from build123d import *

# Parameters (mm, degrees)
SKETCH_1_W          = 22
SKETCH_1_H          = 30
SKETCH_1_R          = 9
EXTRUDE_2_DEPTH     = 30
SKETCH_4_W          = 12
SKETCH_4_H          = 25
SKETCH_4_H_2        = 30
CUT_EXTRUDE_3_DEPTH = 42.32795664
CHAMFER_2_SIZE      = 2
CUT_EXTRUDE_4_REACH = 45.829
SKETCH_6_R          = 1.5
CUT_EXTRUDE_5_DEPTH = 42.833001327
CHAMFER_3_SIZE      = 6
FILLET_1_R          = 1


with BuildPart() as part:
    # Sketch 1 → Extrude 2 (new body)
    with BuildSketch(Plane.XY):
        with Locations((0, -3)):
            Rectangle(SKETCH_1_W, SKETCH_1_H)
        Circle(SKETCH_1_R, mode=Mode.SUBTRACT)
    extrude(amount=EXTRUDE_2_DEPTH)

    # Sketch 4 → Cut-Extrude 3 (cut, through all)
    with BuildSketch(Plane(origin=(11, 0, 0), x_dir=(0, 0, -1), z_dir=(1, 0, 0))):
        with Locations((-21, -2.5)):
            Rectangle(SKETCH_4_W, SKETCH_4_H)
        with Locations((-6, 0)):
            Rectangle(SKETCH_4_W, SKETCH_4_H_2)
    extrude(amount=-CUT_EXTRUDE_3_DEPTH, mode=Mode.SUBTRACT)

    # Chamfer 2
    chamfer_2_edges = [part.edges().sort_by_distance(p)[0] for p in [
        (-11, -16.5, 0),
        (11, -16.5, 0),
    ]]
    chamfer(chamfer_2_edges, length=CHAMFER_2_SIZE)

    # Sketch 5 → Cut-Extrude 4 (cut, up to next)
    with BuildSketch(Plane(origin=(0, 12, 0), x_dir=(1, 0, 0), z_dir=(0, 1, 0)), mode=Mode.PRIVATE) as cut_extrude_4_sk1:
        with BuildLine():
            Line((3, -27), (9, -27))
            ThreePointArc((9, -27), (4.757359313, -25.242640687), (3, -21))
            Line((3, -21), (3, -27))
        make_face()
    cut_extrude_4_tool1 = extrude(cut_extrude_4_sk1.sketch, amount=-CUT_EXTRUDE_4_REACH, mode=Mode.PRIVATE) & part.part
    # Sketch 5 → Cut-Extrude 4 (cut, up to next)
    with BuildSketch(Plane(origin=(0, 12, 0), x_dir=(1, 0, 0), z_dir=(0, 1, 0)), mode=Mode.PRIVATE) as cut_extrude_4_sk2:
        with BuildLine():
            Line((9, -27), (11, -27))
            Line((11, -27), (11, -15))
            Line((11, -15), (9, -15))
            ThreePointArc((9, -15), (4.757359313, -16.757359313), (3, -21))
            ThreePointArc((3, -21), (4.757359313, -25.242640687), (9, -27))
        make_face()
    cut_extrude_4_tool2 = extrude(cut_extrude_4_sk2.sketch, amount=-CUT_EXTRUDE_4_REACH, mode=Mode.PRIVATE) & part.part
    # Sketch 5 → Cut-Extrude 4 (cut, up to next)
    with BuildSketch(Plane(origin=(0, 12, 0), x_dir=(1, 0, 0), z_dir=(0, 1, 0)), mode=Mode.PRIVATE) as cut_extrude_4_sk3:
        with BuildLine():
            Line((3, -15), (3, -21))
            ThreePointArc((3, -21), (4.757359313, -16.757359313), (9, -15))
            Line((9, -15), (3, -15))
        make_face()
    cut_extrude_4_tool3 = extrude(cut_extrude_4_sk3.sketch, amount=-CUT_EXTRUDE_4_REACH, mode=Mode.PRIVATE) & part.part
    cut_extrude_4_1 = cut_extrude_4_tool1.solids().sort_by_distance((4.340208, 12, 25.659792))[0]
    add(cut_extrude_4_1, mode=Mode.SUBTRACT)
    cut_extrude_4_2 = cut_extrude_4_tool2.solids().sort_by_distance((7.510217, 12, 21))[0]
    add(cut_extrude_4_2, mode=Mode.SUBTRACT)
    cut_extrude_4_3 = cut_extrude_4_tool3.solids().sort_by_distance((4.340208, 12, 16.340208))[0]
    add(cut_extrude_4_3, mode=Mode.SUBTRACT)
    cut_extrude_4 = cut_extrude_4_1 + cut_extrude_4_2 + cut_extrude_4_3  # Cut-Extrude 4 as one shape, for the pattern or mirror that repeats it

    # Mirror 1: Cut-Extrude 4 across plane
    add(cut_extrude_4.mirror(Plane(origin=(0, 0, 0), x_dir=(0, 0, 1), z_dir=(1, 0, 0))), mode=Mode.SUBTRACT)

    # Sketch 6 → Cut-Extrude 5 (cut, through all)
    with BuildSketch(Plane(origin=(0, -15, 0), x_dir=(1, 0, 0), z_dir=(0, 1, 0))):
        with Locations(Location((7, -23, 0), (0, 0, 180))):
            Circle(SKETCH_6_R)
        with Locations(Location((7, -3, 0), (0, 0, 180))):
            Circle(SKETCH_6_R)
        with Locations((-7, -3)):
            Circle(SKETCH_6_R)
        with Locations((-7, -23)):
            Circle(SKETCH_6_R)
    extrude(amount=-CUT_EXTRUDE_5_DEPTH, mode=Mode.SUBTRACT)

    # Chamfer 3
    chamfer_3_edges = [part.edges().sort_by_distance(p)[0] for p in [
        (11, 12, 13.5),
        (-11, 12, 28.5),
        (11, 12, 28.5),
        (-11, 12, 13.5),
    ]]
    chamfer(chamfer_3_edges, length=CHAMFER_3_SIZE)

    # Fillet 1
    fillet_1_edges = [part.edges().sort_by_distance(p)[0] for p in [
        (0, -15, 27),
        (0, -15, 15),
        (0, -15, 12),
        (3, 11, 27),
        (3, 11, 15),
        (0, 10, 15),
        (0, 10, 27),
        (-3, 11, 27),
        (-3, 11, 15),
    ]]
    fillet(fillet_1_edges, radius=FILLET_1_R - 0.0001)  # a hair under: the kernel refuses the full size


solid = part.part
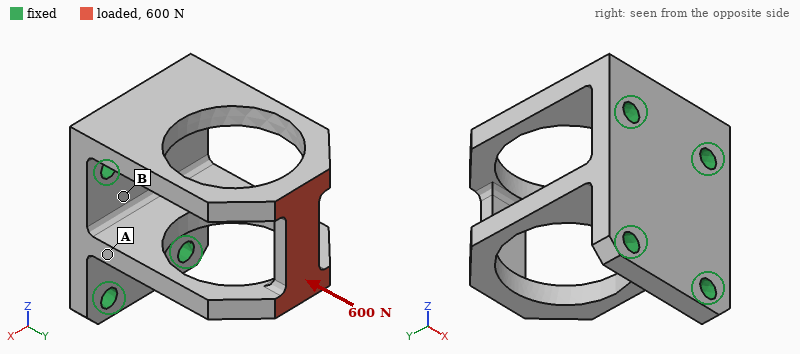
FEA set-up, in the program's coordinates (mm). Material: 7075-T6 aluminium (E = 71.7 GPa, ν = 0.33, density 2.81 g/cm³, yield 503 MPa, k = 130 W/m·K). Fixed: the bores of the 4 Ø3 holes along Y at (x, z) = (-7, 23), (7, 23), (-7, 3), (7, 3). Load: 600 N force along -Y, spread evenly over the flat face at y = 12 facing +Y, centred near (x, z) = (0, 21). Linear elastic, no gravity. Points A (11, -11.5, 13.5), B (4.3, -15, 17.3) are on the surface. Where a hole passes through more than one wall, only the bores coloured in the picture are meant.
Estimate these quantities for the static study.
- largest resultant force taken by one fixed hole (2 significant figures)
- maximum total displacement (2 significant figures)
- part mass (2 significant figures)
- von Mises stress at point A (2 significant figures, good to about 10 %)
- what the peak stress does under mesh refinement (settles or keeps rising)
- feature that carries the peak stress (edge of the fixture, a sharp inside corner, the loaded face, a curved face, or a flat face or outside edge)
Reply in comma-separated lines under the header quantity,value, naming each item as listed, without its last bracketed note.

quantity,value
largest resultant force taken by one fixed hole,230 N
maximum total displacement,65 µm
part mass,11 g
von Mises stress at point A,29 MPa
what the peak stress does under mesh refinement,keeps rising
feature that carries the peak stress,a sharp inside corner
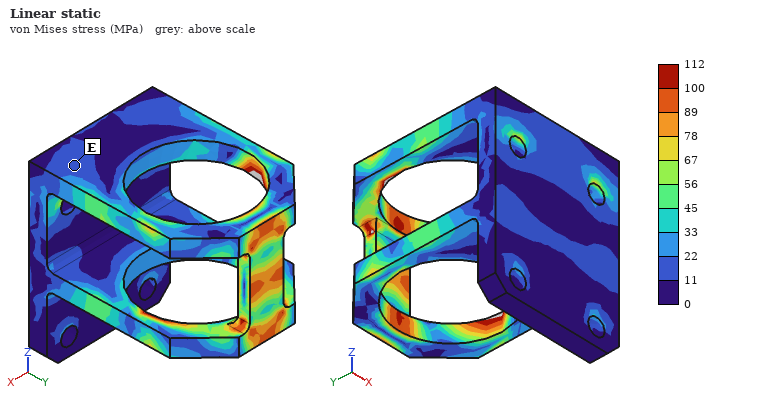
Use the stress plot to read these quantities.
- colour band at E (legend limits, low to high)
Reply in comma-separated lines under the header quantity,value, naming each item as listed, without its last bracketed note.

quantity,value
colour band at E,11 to 22 MPa
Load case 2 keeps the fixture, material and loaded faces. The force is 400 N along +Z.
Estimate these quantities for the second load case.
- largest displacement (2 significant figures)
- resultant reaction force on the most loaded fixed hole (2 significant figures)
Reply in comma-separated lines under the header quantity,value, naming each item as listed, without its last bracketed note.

quantity,value
largest displacement,0.49 mm
resultant reaction force on the most loaded fixed hole,260 N
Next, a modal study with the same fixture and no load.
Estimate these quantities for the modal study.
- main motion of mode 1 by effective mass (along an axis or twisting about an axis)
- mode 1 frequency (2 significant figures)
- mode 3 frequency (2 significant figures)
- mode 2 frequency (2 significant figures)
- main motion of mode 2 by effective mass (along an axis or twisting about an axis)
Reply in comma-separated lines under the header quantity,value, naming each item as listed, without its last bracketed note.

quantity,value
main motion of mode 1 by effective mass,along Z
mode 1 frequency,3600 Hz
mode 3 frequency,7900 Hz
mode 2 frequency,6700 Hz
main motion of mode 2 by effective mass,along X
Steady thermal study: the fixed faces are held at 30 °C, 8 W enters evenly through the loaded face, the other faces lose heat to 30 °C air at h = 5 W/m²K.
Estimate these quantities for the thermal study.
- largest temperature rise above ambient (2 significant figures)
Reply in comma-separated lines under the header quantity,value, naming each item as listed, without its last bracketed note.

quantity,value
largest temperature rise above ambient,51 K
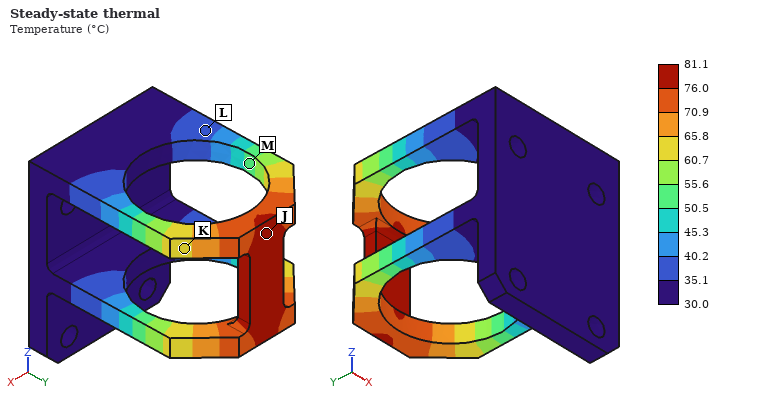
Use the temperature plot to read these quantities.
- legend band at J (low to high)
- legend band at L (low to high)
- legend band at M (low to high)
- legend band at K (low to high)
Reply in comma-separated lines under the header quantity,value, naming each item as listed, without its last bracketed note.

quantity,value
legend band at J,76.0 to 81.1 °C
legend band at L,35.1 to 40.2 °C
legend band at M,50.5 to 55.6 °C
legend band at K,60.7 to 65.8 °C
